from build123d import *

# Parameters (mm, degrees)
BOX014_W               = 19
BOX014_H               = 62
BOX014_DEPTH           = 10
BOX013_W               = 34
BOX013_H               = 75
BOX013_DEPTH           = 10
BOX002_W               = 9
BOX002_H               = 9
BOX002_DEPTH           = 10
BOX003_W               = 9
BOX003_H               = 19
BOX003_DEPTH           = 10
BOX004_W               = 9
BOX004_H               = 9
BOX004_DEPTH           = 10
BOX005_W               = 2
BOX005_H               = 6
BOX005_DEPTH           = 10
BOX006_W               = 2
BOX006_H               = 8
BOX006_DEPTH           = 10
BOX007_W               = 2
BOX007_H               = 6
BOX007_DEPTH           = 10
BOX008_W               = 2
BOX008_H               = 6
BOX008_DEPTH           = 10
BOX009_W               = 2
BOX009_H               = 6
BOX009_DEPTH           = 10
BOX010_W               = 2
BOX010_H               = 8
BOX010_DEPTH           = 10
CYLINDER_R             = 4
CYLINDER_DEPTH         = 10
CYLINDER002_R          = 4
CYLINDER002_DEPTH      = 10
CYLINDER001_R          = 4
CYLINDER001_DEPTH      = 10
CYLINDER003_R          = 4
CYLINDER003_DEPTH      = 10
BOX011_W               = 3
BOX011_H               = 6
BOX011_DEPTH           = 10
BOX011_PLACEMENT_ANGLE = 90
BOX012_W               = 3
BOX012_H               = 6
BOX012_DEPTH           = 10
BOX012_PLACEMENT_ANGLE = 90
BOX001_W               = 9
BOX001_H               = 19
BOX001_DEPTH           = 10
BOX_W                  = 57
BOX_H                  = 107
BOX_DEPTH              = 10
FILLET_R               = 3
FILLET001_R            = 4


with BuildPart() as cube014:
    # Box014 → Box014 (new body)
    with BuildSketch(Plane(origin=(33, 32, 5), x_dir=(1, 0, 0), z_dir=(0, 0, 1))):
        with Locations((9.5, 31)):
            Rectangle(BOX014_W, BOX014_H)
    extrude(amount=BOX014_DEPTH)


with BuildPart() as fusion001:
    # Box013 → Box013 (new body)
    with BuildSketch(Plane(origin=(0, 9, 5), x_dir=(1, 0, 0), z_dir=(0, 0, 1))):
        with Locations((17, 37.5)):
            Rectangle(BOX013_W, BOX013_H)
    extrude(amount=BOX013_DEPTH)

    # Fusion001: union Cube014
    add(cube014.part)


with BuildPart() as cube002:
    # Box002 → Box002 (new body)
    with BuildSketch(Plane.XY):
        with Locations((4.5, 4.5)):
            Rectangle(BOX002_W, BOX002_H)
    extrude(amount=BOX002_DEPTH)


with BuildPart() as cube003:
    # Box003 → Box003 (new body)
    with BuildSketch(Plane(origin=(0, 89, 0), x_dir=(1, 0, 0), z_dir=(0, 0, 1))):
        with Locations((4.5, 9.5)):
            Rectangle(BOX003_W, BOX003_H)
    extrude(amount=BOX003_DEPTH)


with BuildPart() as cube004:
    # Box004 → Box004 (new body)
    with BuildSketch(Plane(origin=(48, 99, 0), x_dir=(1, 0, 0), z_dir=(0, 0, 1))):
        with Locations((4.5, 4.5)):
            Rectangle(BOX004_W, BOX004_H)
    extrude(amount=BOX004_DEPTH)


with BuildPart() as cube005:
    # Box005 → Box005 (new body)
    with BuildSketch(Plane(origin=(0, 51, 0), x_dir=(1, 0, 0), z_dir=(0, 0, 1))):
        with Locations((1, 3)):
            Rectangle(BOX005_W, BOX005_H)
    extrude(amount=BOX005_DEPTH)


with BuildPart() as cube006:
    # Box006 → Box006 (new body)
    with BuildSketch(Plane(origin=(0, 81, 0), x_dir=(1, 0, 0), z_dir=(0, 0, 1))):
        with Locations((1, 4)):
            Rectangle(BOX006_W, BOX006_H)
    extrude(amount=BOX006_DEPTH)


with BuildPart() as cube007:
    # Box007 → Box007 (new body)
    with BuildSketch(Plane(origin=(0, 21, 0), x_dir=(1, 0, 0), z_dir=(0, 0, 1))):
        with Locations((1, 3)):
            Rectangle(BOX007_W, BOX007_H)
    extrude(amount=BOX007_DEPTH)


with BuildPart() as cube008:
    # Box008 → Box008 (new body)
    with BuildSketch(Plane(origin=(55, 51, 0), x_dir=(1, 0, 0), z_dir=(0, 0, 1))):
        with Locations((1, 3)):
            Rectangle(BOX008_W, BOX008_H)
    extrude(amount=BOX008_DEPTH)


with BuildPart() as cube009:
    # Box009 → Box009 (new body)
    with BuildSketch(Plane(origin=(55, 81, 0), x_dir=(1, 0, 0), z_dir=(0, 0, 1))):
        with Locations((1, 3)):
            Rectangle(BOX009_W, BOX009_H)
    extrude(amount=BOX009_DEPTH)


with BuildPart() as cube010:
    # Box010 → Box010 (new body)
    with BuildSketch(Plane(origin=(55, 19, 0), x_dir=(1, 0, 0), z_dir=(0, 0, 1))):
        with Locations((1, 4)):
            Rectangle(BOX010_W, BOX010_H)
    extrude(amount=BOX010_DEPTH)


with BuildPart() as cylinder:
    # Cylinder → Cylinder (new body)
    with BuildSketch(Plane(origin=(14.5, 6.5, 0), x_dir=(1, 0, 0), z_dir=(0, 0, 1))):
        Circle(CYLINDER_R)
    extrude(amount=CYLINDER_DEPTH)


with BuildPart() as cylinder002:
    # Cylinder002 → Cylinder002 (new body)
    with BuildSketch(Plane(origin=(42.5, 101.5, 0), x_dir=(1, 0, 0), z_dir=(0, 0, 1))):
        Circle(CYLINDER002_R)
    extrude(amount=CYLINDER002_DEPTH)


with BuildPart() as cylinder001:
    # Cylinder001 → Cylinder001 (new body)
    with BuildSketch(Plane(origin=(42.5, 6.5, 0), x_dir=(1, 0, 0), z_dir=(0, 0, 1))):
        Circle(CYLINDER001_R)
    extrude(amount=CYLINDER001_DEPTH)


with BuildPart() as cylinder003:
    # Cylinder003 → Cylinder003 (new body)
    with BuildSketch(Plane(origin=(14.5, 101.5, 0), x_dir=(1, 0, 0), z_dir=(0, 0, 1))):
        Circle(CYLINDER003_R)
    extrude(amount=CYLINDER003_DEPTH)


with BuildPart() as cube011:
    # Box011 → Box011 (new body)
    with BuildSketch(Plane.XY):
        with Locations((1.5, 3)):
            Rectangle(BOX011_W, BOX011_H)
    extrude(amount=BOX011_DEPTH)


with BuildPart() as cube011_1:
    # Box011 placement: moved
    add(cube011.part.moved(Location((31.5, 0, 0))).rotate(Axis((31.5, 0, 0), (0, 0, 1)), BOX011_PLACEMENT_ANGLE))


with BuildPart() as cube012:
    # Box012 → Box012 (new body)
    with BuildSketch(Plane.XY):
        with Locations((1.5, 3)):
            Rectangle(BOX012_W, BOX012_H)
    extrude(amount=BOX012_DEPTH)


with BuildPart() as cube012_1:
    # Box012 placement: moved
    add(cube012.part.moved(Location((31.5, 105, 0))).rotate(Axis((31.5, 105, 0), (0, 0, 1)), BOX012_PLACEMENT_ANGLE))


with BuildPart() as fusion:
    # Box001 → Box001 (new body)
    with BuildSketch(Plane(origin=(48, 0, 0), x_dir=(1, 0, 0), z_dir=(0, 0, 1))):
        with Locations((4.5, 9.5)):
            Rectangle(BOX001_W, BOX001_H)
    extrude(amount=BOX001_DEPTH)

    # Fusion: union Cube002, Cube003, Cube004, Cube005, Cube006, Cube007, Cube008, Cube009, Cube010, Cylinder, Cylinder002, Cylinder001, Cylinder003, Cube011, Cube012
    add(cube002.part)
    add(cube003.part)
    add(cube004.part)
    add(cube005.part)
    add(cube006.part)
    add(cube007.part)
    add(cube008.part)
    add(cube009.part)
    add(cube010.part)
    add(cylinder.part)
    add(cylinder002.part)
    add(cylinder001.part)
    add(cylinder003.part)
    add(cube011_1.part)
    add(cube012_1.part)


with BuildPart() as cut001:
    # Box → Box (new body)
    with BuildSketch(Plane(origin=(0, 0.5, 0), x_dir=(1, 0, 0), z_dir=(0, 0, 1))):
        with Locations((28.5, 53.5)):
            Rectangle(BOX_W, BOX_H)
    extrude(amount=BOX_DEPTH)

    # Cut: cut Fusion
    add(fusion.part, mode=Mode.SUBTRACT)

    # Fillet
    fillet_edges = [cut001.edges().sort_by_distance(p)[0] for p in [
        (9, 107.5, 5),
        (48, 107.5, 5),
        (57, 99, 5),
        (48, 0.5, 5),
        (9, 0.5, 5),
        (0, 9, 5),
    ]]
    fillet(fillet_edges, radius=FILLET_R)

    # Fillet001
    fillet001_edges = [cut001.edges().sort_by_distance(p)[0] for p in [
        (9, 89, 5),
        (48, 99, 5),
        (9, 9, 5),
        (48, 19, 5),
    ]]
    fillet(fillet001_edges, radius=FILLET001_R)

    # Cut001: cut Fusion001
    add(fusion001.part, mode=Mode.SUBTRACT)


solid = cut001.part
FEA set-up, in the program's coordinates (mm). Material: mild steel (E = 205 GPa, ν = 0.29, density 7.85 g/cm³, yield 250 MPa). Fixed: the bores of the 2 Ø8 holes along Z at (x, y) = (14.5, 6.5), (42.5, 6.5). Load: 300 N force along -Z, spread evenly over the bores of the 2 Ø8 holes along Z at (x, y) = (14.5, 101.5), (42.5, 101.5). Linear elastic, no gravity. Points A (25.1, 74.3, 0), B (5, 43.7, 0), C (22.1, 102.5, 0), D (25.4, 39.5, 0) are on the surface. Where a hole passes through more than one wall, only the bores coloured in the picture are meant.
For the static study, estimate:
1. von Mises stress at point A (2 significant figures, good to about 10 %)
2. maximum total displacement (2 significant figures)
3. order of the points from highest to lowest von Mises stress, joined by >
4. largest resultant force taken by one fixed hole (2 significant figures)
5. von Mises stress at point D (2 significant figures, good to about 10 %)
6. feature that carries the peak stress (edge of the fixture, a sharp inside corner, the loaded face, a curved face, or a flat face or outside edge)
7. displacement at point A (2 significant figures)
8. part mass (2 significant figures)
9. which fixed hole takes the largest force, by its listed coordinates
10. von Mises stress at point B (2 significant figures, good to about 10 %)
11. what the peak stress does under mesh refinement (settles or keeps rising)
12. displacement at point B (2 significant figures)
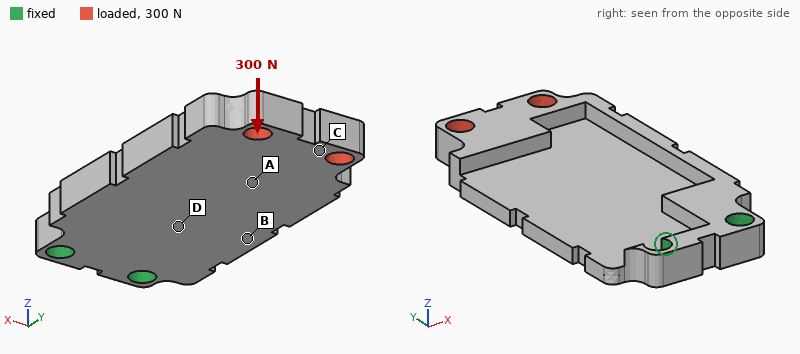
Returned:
22 MPa
0.37 mm
D > B > A > C
400 N
49 MPa
a sharp inside corner
0.18 mm
270 g
(42.5, 6.5)
37 MPa
keeps rising
0.062 mm
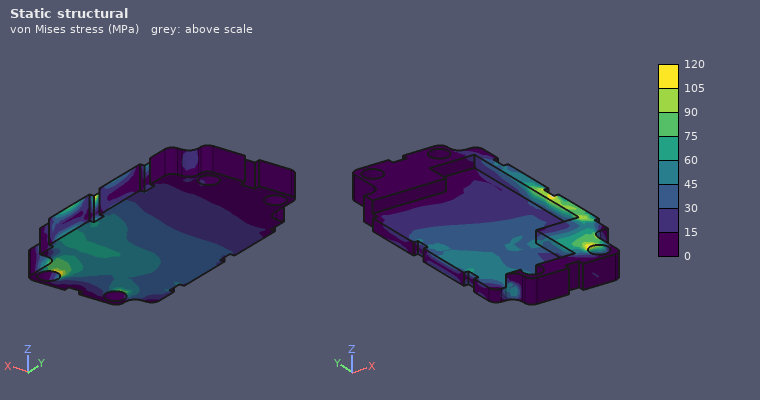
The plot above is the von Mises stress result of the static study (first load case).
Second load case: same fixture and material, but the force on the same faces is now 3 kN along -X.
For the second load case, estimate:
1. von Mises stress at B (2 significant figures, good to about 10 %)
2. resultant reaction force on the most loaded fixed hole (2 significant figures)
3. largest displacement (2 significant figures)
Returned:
50 MPa
9.0 kN
0.20 mm
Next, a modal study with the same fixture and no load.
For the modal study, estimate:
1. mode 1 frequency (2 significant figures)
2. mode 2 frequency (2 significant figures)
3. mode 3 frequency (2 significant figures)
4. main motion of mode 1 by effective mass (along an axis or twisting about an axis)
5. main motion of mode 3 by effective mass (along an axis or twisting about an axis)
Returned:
560 Hz
1800 Hz
3000 Hz
along Z
along X
